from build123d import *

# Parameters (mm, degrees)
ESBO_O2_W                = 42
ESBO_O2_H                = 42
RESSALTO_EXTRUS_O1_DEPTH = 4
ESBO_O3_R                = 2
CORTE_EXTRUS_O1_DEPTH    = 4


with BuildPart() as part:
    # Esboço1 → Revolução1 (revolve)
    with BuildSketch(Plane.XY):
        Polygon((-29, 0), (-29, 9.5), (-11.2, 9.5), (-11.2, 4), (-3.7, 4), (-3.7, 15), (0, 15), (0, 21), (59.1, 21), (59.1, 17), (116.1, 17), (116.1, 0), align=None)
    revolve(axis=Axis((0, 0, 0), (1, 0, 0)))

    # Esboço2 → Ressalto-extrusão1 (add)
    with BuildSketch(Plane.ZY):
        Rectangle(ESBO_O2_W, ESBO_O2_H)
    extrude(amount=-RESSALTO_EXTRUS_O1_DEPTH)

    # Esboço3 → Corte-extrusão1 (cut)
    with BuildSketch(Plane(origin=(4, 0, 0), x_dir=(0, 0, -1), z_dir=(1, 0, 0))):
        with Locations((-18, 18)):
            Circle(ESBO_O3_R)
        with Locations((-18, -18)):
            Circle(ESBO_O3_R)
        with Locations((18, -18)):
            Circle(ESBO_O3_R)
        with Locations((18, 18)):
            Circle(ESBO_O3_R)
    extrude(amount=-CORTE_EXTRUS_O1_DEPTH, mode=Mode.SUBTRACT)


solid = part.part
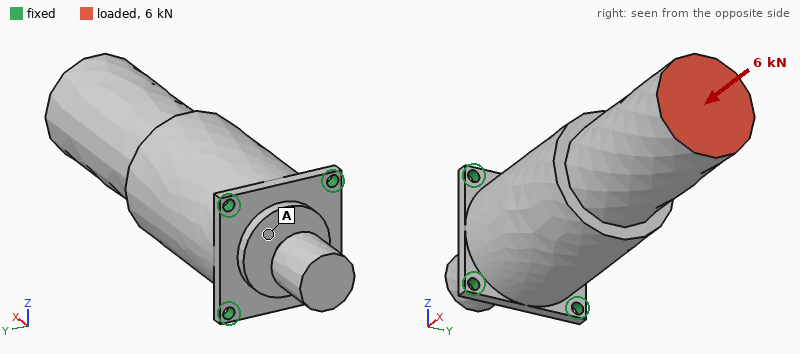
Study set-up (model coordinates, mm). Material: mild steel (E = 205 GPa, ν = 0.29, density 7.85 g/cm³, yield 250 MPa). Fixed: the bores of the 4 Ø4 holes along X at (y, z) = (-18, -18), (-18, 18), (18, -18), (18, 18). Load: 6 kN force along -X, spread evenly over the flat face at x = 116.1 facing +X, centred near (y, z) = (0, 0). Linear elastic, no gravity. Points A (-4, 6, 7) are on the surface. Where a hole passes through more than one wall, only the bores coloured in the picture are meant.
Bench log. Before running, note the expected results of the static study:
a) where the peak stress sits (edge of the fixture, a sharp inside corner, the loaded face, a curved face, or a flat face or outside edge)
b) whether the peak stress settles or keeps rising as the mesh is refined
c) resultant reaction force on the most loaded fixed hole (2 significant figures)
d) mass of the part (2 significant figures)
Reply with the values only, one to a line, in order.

edge of the fixture
keeps rising
1.6 kN
1.1 kg
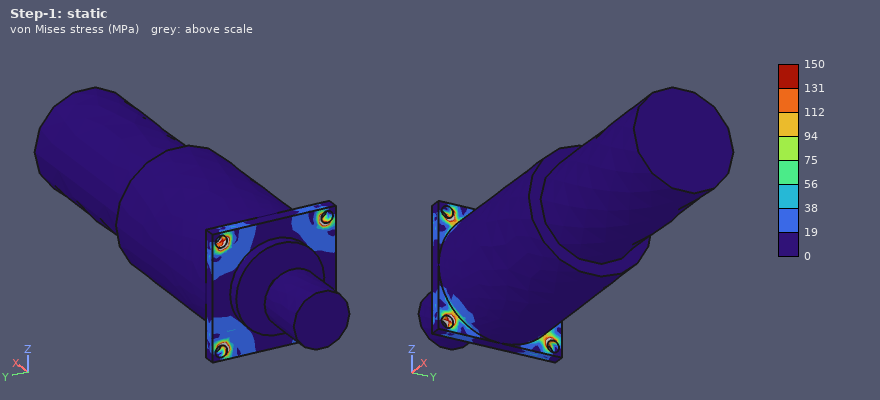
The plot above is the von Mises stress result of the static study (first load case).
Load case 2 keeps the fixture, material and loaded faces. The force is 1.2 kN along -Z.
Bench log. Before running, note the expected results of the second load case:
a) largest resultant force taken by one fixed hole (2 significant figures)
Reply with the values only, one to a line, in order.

2.2 kN
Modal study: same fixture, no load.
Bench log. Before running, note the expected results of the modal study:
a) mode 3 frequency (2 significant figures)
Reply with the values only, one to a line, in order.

3200 Hz
